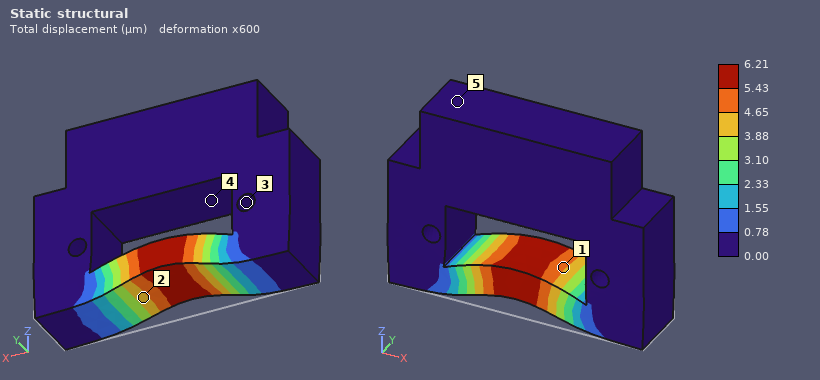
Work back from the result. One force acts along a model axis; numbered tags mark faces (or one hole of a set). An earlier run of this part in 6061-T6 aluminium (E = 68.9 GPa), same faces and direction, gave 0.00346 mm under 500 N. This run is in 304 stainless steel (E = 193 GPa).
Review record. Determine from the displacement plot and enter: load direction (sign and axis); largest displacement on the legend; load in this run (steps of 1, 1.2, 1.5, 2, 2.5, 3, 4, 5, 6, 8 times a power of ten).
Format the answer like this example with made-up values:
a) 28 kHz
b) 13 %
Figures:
a) +Z
b) 6.21 µm
c) 2.5 kN
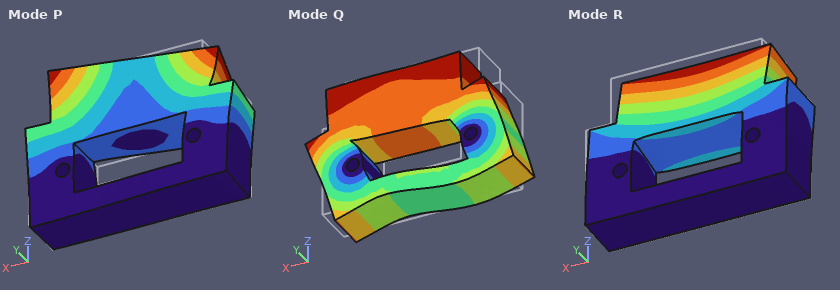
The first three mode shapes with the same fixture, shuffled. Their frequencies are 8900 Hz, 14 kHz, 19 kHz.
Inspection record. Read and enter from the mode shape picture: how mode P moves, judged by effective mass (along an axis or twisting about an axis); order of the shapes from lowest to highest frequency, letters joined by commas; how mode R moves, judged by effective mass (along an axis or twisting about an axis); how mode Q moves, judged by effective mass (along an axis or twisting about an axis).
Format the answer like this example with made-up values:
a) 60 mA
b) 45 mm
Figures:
a) twisting about Z
b) R, Q, P
c) along Y
d) along X
